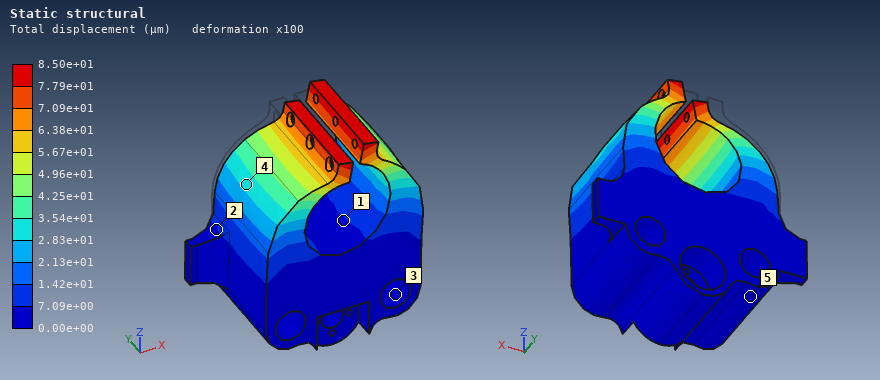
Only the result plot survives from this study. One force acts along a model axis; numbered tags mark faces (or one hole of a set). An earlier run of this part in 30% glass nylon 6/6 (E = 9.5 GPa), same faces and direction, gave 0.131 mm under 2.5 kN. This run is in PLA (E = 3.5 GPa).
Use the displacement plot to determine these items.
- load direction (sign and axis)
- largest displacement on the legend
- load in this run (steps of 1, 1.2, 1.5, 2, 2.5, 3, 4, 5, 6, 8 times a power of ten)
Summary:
+X
8.50e+01 µm
600 N
